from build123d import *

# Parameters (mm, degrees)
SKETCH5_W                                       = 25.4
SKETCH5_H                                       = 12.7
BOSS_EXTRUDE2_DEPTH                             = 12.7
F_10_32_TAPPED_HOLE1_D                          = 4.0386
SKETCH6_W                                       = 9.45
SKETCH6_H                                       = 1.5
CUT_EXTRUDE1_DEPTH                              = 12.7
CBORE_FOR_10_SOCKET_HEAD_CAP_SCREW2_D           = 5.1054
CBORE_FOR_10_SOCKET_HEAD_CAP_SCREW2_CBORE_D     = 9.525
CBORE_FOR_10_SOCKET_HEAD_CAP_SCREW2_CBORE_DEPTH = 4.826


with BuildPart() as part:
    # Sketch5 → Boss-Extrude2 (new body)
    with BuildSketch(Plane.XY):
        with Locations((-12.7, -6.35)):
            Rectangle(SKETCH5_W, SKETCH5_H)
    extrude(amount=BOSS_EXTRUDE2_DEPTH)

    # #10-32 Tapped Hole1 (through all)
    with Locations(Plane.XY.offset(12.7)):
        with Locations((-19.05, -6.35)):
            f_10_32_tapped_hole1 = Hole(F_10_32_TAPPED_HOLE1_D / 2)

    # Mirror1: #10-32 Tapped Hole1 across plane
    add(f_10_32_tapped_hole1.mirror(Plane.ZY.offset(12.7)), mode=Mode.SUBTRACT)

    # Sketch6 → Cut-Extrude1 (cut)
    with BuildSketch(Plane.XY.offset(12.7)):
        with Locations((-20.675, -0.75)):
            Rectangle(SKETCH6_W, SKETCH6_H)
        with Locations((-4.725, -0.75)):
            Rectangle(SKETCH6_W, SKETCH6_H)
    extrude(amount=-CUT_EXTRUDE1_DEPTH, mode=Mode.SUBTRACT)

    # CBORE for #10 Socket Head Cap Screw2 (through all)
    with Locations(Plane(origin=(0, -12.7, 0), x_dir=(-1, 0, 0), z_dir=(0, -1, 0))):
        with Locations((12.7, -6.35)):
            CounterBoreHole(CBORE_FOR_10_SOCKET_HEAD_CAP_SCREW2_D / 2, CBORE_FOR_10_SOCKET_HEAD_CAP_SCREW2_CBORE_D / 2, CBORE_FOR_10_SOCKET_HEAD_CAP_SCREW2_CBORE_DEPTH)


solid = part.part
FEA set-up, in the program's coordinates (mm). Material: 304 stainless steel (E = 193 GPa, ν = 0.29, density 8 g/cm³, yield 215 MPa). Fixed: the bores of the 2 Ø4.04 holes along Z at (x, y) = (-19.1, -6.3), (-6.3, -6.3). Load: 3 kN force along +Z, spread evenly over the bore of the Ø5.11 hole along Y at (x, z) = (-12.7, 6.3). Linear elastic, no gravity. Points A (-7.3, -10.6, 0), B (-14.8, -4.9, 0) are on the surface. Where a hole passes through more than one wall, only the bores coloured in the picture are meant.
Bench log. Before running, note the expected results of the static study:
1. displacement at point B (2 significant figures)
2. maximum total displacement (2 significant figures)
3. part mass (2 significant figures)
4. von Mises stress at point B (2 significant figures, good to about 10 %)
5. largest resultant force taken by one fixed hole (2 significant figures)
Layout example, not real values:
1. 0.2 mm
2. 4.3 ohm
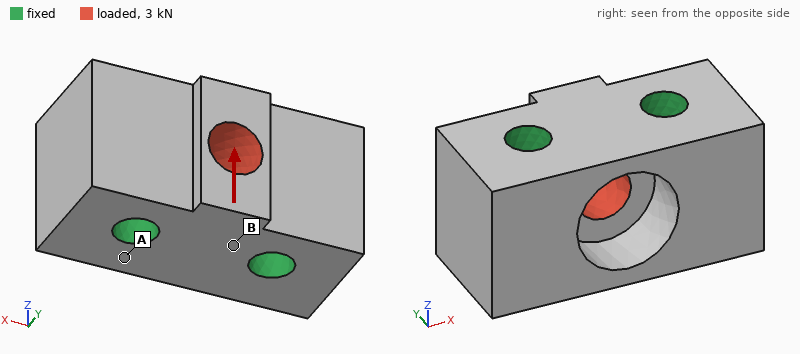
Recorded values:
1. 0.79 µm
2. 2.0 µm
3. 23 g
4. 15 MPa
5. 1.5 kN
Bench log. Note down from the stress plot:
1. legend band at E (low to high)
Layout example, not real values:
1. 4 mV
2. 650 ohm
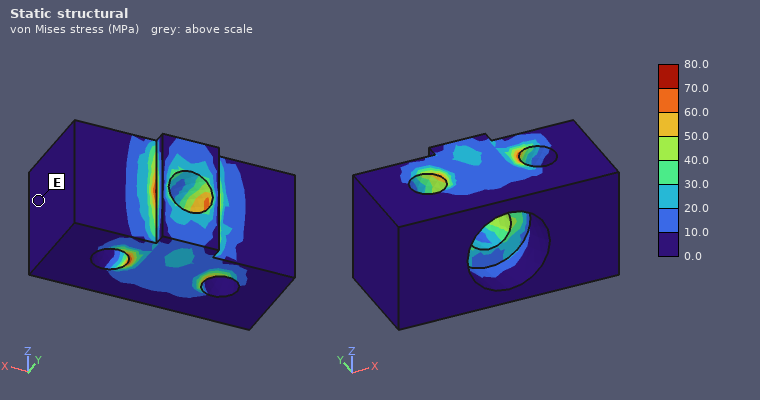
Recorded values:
1. 0.0 to 10.0 MPa
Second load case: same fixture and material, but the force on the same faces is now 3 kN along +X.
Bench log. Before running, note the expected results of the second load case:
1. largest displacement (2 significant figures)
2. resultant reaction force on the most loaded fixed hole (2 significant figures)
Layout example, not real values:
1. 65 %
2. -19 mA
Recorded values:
1. 2.6 µm
2. 1.5 kN
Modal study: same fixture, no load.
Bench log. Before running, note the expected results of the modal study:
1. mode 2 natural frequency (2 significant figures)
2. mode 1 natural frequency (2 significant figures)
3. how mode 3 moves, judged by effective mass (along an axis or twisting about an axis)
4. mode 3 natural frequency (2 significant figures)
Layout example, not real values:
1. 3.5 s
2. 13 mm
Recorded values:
1. 80 kHz
2. 80 kHz
3. along Z
4. 100 kHz
